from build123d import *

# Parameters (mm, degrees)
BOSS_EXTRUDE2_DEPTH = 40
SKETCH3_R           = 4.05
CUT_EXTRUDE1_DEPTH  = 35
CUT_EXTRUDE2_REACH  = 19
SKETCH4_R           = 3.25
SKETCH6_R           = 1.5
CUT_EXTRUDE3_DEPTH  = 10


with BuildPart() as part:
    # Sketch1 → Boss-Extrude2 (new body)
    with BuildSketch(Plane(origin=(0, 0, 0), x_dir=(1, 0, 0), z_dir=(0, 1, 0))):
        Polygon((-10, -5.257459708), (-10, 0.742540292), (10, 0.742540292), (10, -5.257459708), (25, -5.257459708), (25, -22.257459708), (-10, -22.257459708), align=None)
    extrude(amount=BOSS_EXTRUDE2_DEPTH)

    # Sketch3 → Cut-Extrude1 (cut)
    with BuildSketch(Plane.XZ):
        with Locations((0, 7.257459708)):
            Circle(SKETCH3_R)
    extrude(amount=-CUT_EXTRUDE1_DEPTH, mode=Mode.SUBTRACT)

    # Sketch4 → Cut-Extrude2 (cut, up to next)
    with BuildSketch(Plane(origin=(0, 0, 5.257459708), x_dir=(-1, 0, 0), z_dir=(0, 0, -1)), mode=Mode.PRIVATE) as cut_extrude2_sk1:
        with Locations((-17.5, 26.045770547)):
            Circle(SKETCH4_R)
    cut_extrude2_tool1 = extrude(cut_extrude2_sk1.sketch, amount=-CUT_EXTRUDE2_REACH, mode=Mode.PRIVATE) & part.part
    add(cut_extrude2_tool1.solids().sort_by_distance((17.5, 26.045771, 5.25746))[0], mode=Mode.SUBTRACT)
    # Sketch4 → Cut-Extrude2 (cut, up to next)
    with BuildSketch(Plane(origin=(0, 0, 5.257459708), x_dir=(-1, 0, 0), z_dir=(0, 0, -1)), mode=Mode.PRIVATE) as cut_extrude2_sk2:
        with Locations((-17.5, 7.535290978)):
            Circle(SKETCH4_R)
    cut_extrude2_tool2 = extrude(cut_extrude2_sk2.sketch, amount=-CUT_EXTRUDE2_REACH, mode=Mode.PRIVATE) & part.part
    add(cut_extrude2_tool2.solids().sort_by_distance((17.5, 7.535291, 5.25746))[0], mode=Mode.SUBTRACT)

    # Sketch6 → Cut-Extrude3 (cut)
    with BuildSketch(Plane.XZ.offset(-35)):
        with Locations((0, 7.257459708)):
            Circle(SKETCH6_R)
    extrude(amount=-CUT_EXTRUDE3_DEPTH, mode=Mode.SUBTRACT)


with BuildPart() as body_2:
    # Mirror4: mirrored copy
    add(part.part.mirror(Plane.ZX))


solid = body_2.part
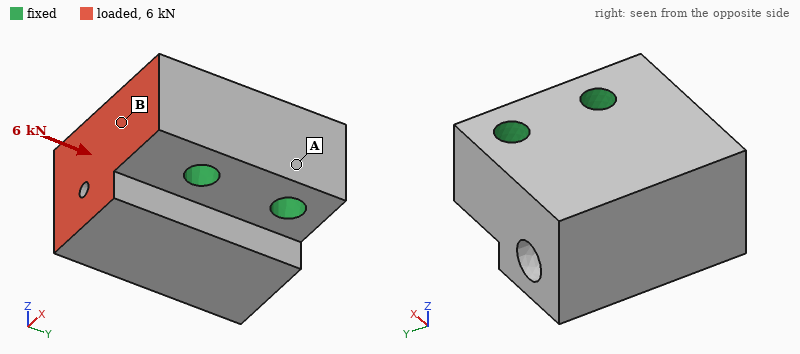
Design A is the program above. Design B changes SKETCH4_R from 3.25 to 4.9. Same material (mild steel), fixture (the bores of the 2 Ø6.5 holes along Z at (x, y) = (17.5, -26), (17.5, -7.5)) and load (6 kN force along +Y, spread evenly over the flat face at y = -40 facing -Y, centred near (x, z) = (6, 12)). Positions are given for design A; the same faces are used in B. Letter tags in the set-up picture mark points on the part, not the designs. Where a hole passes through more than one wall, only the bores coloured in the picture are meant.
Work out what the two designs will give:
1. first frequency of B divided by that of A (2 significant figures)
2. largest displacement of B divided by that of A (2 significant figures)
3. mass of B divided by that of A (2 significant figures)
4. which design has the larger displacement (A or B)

1.2
0.80
0.94
A
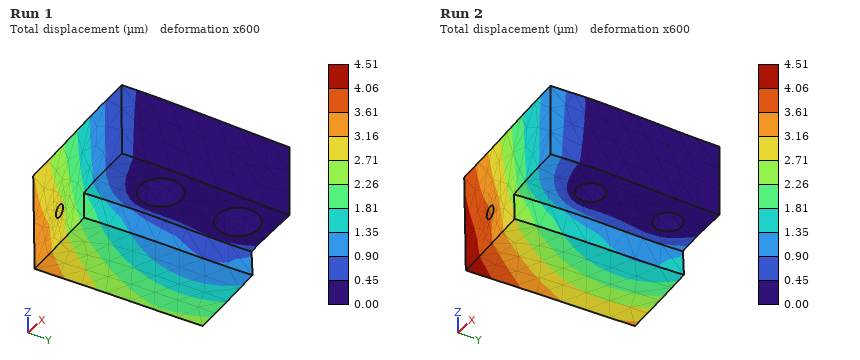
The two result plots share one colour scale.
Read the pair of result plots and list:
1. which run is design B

Run 1
